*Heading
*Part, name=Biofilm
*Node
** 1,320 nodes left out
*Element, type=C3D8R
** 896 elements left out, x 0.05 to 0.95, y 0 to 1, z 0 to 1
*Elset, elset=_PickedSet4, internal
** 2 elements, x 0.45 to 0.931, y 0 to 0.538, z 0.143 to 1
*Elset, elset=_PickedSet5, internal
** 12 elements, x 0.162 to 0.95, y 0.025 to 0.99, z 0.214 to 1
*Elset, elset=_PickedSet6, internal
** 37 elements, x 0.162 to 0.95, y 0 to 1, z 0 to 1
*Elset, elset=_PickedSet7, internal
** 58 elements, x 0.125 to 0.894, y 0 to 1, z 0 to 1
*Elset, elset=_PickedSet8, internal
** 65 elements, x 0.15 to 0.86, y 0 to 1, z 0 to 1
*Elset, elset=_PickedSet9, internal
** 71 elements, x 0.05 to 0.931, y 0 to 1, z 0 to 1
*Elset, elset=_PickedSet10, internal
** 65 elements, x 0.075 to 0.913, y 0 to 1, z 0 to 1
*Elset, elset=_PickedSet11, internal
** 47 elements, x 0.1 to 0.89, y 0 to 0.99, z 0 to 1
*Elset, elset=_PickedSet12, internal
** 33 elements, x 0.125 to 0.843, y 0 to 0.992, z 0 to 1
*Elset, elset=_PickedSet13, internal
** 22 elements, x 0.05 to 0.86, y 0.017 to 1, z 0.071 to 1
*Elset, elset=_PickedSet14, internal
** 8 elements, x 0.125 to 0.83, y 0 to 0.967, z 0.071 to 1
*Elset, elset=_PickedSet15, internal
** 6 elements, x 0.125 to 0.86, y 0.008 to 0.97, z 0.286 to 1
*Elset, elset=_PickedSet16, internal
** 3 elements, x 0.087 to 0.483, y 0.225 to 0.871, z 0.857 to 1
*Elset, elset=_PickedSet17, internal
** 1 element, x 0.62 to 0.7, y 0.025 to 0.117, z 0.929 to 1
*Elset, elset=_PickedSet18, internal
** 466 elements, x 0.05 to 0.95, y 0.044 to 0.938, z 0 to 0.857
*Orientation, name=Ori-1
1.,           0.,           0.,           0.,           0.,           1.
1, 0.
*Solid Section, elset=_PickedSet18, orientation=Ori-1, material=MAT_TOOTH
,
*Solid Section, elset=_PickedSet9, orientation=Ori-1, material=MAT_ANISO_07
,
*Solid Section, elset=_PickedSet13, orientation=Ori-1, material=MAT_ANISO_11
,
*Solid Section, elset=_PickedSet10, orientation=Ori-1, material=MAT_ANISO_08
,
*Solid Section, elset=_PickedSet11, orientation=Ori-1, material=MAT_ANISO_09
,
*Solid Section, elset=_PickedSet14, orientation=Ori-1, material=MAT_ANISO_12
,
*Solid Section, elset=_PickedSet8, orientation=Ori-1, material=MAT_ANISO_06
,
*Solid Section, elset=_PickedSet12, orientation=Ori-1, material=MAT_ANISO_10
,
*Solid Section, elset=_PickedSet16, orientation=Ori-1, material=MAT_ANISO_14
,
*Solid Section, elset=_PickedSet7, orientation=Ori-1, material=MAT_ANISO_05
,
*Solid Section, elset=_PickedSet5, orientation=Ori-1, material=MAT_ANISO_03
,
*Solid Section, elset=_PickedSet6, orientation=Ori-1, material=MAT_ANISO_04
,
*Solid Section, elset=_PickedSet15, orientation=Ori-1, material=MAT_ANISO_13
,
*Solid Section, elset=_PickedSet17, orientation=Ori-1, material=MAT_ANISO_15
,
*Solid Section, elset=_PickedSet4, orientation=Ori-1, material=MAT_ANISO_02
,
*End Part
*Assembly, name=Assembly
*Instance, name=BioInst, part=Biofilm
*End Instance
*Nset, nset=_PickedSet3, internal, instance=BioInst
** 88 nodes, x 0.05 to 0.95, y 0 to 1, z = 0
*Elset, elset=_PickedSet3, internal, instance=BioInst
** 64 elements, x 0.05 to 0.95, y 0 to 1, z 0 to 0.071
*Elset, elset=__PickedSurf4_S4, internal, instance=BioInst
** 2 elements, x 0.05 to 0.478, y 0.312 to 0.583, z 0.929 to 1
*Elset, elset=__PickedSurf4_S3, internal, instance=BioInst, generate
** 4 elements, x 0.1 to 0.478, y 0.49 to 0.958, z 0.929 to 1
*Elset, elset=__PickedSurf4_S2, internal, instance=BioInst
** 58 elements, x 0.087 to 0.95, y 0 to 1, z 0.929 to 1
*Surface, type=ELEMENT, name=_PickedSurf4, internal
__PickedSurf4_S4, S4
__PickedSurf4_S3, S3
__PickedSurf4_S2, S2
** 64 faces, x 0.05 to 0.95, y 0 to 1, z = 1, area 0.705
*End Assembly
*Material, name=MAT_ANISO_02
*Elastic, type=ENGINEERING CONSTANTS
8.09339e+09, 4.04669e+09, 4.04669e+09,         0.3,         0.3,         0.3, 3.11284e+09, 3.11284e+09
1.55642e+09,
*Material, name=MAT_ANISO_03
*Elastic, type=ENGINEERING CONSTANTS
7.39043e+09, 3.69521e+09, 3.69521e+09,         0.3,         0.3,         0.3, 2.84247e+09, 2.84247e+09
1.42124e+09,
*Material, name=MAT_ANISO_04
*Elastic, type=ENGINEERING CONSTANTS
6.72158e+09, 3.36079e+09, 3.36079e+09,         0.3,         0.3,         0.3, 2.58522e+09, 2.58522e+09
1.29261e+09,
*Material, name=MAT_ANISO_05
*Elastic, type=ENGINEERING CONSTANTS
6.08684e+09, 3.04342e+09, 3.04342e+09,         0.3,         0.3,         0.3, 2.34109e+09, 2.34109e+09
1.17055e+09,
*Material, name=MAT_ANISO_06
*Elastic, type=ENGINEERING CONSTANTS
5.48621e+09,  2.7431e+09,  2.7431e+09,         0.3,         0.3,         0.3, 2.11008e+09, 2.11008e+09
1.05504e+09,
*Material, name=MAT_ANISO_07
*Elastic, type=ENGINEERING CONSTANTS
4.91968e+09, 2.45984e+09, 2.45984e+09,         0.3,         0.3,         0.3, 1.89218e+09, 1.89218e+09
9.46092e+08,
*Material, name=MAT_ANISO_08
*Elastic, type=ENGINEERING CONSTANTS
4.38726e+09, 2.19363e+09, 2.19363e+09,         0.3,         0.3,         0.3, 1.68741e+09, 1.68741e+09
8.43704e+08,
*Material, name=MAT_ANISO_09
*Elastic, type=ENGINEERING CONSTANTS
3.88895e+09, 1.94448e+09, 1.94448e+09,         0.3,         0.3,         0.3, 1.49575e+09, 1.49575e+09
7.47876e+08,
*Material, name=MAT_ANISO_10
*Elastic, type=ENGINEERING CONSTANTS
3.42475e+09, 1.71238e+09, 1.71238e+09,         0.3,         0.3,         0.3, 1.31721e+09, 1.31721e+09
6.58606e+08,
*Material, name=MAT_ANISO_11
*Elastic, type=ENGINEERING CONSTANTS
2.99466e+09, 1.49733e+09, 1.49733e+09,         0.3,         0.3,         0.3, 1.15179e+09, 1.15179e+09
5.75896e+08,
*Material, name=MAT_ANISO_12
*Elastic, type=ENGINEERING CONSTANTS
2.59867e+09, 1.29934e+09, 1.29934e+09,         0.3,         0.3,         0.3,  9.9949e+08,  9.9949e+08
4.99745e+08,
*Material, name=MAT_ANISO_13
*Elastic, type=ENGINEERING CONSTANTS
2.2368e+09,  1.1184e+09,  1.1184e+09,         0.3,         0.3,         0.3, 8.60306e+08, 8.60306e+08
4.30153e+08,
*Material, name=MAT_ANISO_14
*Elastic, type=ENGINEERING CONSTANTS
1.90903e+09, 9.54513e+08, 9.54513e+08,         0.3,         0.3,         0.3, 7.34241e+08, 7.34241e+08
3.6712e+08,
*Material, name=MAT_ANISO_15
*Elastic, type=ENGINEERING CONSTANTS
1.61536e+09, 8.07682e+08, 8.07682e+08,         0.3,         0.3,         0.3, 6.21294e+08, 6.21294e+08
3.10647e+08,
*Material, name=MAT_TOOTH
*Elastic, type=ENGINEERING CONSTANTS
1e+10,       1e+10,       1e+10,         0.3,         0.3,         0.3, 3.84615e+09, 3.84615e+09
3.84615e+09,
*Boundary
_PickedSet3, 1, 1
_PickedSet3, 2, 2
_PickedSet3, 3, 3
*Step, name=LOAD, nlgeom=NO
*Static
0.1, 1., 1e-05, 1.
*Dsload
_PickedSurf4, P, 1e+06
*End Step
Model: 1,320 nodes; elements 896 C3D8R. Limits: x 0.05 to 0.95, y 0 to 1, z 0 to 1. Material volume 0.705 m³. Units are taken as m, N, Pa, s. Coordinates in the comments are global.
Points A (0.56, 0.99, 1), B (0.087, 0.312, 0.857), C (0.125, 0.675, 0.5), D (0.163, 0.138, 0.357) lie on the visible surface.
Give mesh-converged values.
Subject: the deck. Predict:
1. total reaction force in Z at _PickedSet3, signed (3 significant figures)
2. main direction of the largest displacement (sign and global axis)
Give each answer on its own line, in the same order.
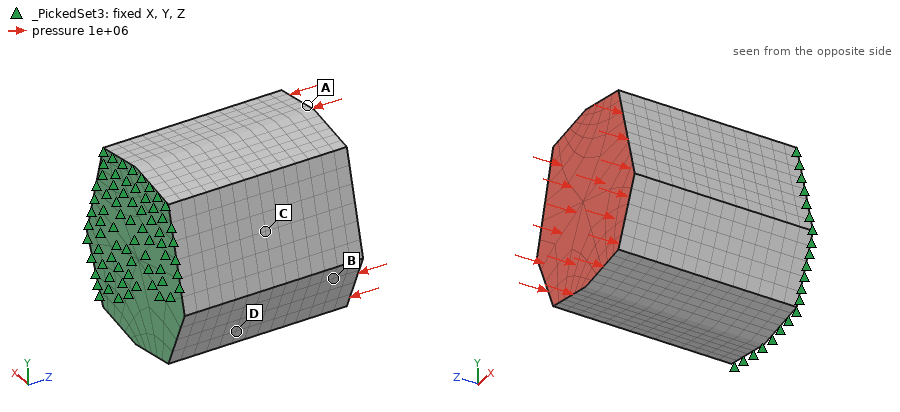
7.05e+05 N
-Z
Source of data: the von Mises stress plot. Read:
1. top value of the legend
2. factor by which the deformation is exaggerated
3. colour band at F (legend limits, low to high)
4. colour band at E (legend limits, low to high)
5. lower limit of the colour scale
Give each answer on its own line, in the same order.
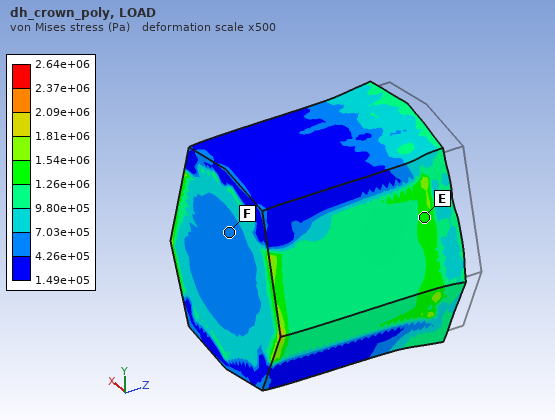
2.64e+06 Pa
500
4.26e+05 to 7.03e+05 Pa
1.26e+06 to 1.54e+06 Pa
1.49e+05 Pa
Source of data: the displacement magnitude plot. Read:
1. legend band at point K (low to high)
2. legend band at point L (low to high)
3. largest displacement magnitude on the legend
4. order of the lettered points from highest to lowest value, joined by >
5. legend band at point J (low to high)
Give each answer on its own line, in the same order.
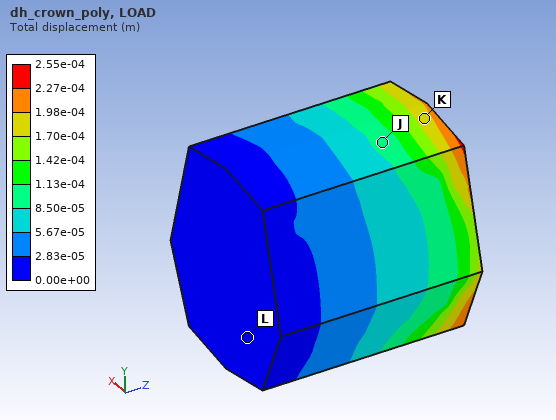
1.70e-04 to 1.98e-04 m
0.00e+00 to 2.83e-05 m
2.55e-04 m
K > J > L
8.50e-05 to 1.13e-04 m
